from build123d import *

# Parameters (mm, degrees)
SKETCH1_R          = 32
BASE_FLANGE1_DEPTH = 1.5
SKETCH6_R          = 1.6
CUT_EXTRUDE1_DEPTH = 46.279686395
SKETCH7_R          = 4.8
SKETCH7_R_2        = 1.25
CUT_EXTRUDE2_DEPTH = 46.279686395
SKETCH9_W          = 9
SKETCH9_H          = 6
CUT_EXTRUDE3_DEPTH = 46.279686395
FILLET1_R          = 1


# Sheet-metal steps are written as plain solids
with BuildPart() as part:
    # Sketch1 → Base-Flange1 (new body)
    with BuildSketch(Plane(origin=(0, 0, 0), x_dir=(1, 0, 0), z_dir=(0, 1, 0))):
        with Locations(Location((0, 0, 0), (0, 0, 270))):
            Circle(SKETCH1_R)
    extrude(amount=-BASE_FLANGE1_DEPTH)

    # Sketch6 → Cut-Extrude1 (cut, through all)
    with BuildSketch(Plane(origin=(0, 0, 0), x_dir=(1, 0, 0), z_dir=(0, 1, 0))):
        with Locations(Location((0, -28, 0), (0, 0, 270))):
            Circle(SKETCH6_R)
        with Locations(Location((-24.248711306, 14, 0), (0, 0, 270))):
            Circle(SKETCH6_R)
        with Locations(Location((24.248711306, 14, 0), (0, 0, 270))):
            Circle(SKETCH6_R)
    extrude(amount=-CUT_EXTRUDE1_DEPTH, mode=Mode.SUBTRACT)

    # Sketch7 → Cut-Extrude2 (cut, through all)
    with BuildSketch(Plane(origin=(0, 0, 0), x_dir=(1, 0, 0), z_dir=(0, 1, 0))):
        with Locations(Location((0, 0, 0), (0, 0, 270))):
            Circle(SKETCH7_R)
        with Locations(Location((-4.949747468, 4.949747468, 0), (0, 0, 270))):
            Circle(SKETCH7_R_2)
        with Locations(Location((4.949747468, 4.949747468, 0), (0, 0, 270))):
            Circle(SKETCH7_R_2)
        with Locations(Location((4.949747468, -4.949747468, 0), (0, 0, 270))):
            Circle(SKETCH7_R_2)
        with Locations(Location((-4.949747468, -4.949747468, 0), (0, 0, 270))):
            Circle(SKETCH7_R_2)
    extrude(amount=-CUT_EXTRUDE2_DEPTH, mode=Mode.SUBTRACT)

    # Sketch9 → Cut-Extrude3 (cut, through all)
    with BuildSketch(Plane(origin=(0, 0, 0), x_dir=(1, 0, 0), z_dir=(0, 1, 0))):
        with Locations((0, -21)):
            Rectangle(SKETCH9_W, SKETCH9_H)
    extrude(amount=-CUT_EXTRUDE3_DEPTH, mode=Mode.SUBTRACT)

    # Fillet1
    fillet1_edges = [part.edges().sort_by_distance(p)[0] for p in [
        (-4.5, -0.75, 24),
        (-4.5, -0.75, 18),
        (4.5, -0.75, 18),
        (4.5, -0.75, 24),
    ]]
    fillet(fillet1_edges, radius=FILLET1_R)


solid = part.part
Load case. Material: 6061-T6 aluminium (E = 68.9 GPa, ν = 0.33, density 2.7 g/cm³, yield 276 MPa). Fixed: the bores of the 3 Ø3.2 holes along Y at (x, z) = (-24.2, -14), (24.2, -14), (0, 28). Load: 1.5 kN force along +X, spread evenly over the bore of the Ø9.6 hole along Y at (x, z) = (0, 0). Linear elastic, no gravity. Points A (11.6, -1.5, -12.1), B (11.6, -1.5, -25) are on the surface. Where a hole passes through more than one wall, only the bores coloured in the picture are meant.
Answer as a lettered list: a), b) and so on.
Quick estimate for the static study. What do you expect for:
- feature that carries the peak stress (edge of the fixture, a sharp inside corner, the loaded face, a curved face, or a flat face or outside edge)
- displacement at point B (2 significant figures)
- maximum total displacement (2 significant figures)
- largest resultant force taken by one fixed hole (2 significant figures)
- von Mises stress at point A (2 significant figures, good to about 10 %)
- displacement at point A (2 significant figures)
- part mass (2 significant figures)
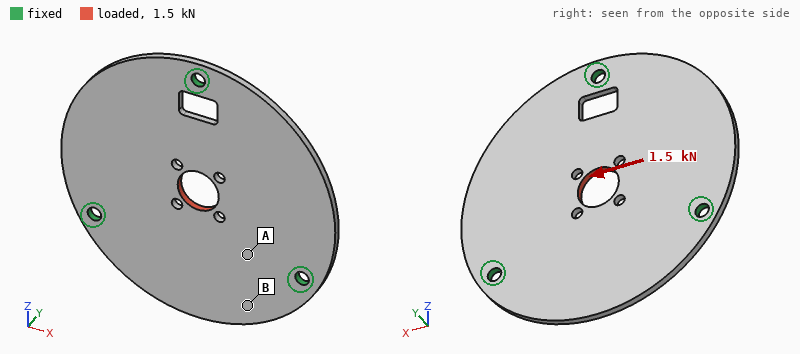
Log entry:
a) a curved face
b) 3.3 µm
c) 15 µm
d) 550 N
e) 21 MPa
f) 4.9 µm
g) 12 g
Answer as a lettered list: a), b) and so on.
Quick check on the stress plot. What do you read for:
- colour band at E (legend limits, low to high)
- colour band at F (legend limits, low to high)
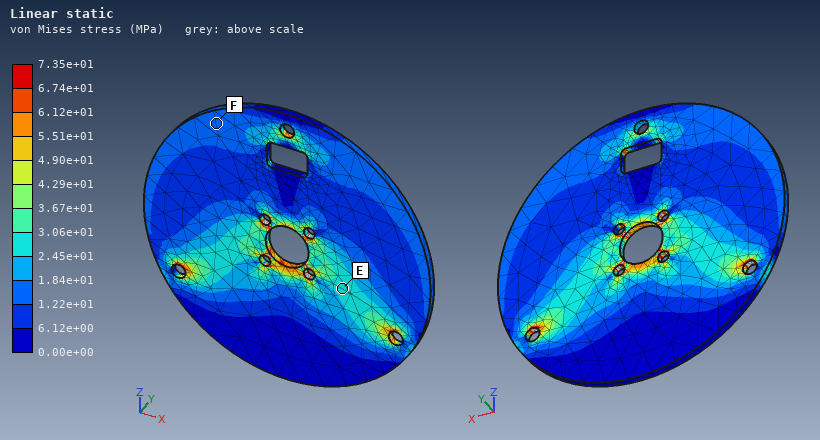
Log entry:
a) 2.45e+01 to 3.06e+01 MPa
b) 1.22e+01 to 1.84e+01 MPa
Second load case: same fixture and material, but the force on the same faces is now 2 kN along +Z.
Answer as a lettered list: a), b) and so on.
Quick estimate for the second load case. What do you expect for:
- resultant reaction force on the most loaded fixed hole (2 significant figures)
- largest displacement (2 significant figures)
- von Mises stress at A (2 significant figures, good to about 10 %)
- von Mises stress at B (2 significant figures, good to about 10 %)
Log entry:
a) 790 N
b) 22 µm
c) 22 MPa
d) 20 MPa
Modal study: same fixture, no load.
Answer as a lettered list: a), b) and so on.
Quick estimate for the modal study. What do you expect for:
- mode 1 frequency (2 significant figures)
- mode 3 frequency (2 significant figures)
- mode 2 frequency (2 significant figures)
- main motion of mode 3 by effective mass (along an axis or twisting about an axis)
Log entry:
a) 2400 Hz
b) 2600 Hz
c) 2400 Hz
d) along Y
